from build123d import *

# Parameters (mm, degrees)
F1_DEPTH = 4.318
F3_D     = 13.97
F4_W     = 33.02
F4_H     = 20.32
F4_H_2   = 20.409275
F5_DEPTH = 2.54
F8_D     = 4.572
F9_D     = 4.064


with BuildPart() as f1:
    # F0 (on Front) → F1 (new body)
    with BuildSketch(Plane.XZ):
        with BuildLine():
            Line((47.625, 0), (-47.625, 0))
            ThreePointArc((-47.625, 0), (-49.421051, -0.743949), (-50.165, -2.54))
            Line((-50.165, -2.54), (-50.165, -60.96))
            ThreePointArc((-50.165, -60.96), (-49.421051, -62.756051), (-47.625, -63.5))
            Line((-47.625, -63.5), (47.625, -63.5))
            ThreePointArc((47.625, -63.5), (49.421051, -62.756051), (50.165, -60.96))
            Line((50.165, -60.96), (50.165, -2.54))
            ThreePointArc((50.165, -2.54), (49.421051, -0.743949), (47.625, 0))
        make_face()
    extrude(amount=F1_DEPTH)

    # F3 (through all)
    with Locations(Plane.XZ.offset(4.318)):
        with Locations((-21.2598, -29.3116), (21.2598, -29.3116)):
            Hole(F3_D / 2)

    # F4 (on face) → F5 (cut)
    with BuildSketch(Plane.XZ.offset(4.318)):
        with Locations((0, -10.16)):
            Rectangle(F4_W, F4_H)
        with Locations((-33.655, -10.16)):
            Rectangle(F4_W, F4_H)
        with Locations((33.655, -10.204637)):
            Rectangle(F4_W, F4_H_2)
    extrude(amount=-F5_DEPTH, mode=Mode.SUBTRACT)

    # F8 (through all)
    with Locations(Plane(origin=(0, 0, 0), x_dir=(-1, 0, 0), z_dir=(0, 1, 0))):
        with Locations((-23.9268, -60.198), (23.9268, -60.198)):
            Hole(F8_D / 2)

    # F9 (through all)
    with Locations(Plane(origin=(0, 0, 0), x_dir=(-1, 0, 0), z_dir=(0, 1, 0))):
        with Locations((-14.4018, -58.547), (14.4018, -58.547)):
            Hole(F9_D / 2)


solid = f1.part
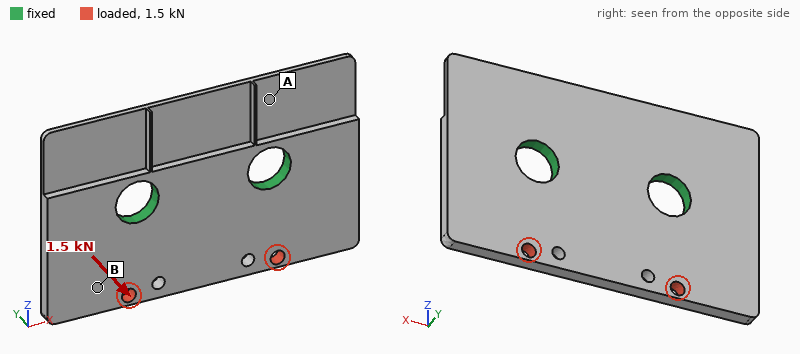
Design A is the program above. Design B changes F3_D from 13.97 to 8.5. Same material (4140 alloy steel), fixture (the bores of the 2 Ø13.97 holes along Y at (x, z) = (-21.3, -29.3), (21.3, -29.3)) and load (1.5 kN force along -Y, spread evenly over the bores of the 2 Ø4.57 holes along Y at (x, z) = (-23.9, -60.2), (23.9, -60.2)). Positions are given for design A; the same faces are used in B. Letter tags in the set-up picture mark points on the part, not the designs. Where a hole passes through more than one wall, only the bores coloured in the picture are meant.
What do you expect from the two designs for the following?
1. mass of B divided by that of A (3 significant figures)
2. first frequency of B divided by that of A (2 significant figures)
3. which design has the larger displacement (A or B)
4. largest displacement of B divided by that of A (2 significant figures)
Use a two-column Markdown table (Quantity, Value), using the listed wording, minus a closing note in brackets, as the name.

| Quantity | Value |
|---|---|
| mass of B divided by that of A | 1.04 |
| first frequency of B divided by that of A | 0.84 |
| which design has the larger displacement | B |
| largest displacement of B divided by that of A | 1.4 |
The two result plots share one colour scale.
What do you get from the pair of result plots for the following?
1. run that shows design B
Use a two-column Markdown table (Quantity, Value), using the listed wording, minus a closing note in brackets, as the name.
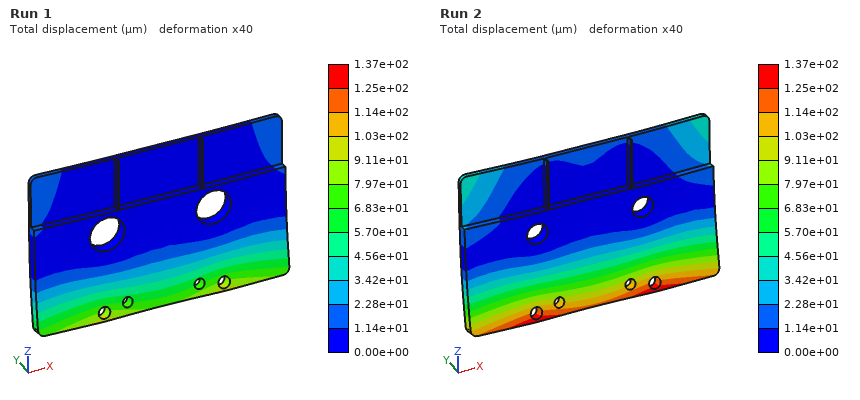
| Quantity | Value |
|---|---|
| run that shows design B | Run 2 |
